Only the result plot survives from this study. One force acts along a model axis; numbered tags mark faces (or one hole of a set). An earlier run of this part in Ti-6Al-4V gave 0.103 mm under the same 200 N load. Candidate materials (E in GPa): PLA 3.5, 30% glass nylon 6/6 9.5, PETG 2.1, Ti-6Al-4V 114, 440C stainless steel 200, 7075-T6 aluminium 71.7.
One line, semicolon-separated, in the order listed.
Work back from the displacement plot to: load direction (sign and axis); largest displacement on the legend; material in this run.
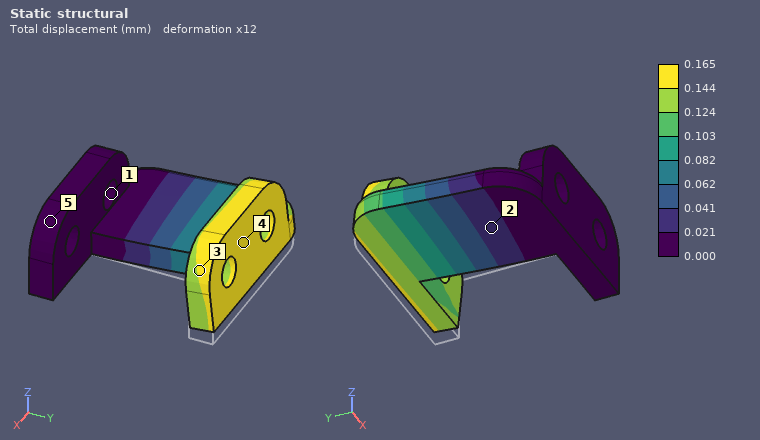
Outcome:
+Z; 0.165 mm; 7075-T6 aluminium
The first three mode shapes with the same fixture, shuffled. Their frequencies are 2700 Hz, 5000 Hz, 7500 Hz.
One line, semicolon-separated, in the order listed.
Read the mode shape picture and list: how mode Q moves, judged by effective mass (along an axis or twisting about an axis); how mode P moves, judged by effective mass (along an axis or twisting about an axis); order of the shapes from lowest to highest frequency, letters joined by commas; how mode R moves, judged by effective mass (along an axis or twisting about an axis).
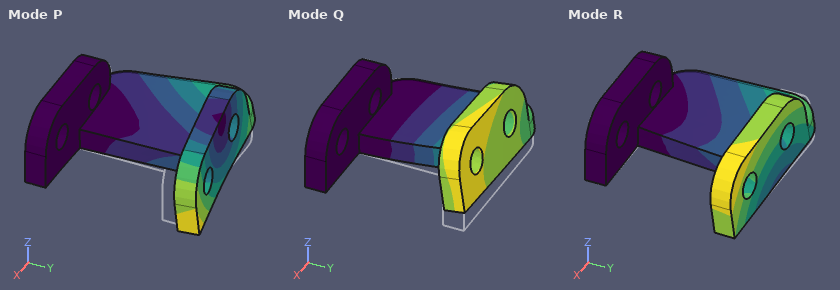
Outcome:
along Z; along X; Q, R, P; along X
